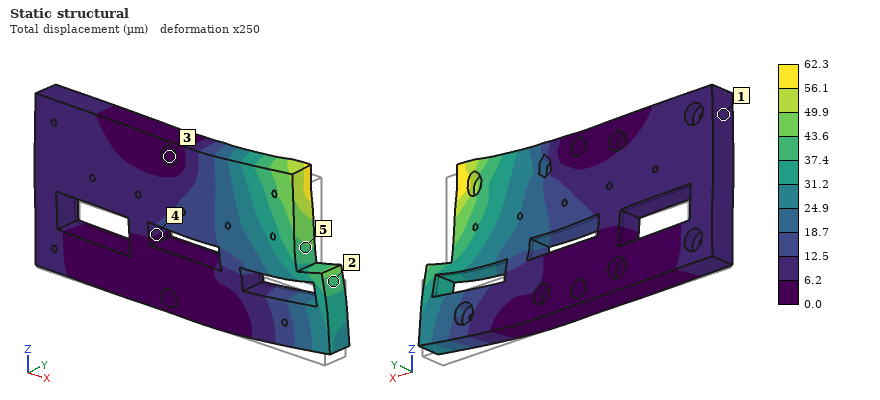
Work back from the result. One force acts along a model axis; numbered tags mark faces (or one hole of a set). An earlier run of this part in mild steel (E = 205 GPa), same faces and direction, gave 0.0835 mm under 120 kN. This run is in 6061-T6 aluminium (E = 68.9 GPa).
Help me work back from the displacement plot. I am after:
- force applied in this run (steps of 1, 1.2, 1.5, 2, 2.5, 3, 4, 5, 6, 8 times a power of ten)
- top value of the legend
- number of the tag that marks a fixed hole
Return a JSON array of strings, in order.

["30 kN", "62.3 µm", "3"]
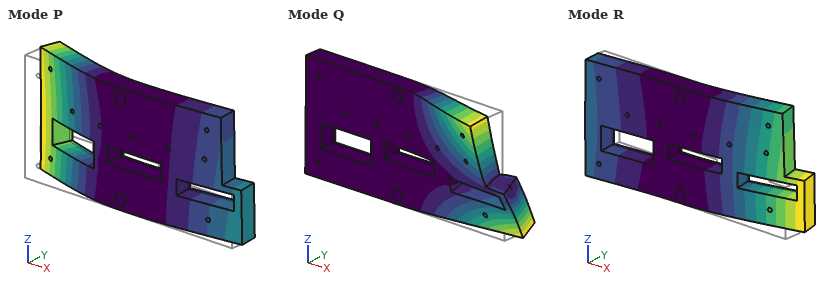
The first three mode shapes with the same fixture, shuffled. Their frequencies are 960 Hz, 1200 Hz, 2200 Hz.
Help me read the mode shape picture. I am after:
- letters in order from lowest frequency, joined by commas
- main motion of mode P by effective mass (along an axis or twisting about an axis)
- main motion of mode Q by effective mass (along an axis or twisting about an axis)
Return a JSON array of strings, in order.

["R, P, Q", "along Y", "twisting about X"]
